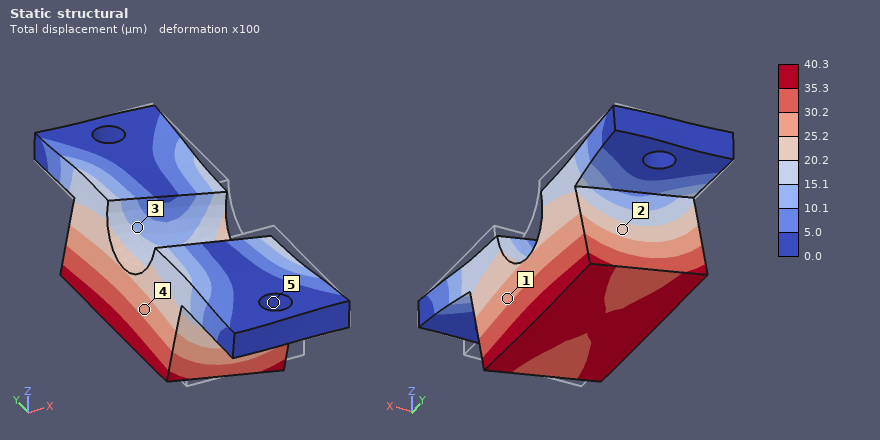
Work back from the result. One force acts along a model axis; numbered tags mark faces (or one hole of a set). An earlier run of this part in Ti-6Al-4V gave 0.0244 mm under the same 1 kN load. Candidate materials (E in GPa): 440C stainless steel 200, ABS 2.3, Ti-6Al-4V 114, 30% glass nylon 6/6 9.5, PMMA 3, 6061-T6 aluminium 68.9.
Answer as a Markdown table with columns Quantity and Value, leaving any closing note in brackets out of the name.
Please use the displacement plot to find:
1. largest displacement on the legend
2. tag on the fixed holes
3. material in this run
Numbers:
| Quantity | Value |
|---|---|
| largest displacement on the legend | 40.3 µm |
| tag on the fixed holes | 5 |
| material in this run | 6061-T6 aluminium |
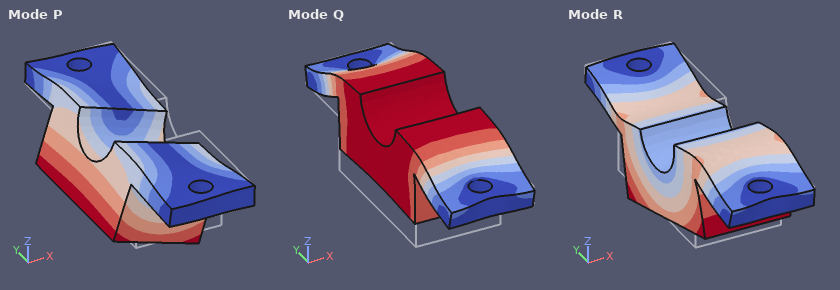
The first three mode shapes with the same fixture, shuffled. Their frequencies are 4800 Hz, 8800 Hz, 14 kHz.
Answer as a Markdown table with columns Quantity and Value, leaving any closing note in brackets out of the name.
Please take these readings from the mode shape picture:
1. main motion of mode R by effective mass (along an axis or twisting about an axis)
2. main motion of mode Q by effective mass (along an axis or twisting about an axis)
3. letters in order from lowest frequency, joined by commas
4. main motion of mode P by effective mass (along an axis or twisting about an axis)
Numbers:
| Quantity | Value |
|---|---|
| main motion of mode R by effective mass | along Y |
| main motion of mode Q by effective mass | along Z |
| letters in order from lowest frequency, joined by commas | P, Q, R |
| main motion of mode P by effective mass | along X |
